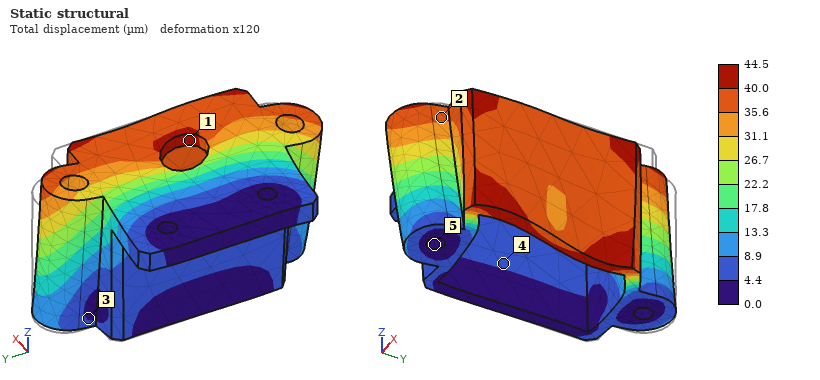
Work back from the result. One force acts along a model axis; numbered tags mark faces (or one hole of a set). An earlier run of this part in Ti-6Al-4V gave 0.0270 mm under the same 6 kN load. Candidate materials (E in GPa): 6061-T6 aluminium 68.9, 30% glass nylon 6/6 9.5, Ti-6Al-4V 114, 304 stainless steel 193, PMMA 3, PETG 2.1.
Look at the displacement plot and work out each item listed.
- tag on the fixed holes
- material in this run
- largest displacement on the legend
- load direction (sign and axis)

5
6061-T6 aluminium
44.5 µm
-Y
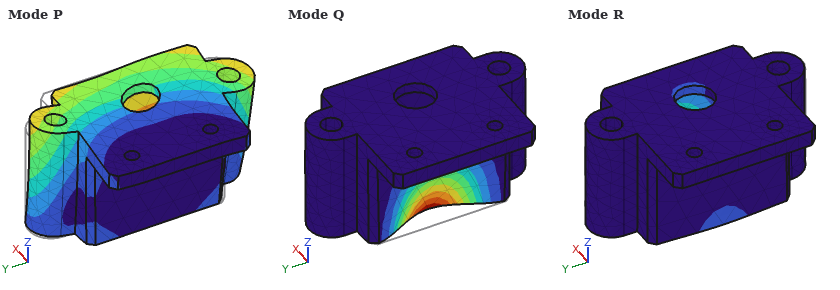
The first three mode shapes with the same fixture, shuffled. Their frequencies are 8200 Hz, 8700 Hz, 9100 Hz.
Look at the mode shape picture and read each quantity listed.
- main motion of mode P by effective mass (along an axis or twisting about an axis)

along Y
